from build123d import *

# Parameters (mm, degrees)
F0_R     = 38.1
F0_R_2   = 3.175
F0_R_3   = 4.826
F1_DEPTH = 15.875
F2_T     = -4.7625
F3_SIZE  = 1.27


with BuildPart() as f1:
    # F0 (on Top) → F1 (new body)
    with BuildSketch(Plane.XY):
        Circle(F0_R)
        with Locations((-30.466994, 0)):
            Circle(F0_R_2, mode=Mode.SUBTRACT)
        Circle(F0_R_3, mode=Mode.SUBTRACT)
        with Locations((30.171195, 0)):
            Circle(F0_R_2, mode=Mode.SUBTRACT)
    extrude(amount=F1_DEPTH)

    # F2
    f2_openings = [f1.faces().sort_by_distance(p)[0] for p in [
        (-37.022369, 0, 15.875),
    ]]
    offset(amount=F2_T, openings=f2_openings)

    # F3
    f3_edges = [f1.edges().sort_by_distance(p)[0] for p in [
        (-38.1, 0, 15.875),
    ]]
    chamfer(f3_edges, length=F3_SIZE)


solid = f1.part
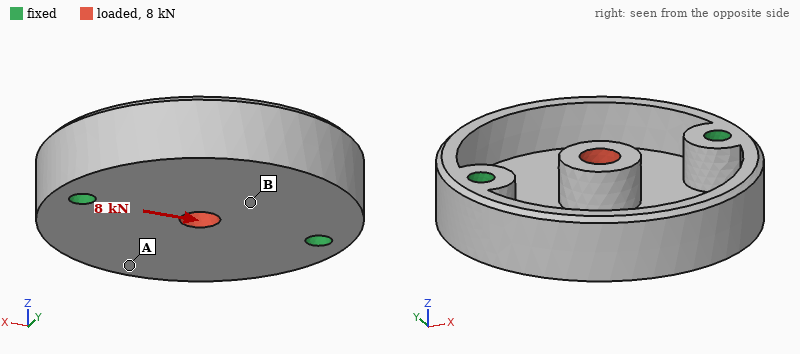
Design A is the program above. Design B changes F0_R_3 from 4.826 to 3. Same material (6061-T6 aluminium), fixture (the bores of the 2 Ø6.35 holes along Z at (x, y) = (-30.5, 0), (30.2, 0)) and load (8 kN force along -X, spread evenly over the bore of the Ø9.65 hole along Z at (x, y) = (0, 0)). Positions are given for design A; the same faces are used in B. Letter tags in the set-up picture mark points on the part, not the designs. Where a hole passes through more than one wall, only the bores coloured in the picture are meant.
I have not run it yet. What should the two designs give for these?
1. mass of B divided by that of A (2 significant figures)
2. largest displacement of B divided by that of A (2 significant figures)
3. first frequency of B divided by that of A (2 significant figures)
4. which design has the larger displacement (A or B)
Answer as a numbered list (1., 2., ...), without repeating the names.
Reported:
1. 0.99
2. 1.3
3. 1.0
4. B
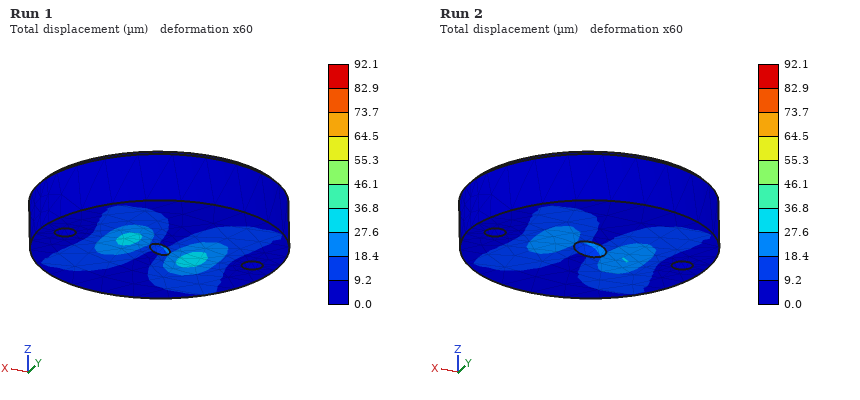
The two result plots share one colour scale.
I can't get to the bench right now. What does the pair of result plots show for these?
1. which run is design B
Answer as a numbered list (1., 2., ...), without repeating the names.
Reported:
1. Run 1
